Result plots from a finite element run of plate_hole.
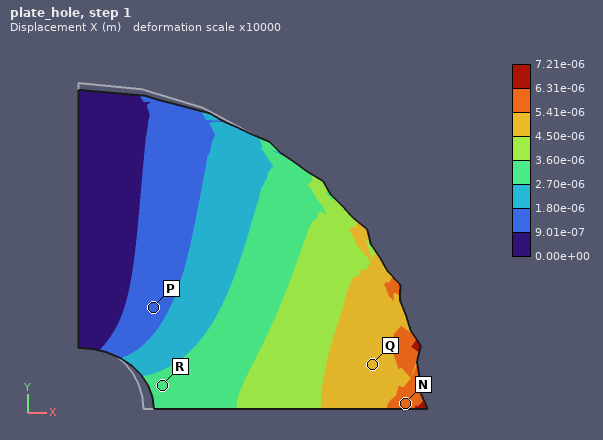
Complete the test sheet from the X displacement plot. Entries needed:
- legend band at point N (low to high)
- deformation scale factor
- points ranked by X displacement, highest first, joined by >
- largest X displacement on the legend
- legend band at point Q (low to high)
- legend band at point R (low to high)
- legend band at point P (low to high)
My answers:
5.41e-06 to 6.31e-06 m
10000
N > Q > R > P
7.21e-06 m
4.50e-06 to 5.41e-06 m
2.70e-06 to 3.60e-06 m
9.01e-07 to 1.80e-06 m
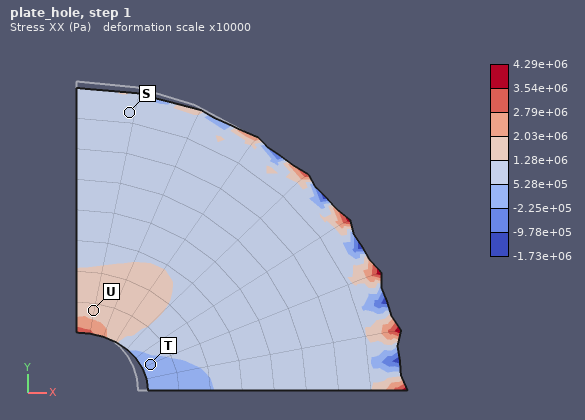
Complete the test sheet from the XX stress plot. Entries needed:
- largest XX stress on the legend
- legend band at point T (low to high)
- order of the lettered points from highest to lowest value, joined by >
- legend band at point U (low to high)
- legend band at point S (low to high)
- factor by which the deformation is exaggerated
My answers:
4.29e+06 Pa
-2.25e+05 to 5.28e+05 Pa
U > S > T
1.28e+06 to 2.03e+06 Pa
5.28e+05 to 1.28e+06 Pa
10000
